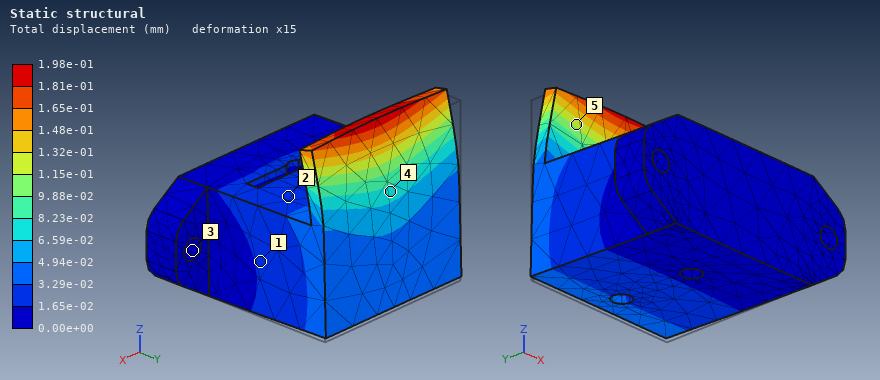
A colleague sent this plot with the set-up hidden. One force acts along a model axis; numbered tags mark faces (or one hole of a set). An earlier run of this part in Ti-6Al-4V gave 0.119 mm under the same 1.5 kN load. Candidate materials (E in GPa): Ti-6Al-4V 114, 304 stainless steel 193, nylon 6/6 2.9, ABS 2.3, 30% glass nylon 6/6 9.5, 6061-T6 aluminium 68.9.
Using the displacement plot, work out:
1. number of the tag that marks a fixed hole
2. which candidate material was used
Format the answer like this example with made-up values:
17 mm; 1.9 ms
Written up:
3; 6061-T6 aluminium
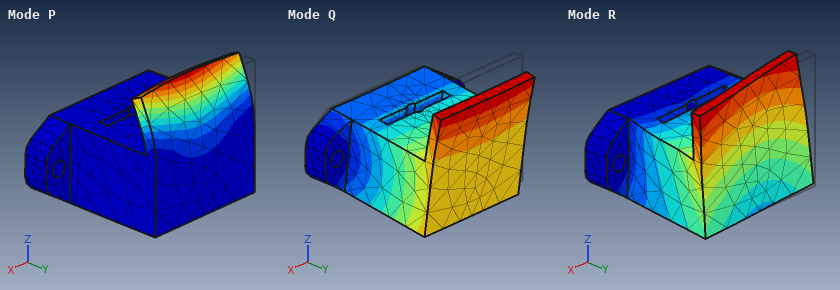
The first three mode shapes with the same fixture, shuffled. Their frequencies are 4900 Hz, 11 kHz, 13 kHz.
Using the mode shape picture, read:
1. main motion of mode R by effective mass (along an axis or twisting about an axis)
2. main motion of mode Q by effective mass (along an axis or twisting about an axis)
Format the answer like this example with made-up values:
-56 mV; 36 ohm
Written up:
along X; along Z
